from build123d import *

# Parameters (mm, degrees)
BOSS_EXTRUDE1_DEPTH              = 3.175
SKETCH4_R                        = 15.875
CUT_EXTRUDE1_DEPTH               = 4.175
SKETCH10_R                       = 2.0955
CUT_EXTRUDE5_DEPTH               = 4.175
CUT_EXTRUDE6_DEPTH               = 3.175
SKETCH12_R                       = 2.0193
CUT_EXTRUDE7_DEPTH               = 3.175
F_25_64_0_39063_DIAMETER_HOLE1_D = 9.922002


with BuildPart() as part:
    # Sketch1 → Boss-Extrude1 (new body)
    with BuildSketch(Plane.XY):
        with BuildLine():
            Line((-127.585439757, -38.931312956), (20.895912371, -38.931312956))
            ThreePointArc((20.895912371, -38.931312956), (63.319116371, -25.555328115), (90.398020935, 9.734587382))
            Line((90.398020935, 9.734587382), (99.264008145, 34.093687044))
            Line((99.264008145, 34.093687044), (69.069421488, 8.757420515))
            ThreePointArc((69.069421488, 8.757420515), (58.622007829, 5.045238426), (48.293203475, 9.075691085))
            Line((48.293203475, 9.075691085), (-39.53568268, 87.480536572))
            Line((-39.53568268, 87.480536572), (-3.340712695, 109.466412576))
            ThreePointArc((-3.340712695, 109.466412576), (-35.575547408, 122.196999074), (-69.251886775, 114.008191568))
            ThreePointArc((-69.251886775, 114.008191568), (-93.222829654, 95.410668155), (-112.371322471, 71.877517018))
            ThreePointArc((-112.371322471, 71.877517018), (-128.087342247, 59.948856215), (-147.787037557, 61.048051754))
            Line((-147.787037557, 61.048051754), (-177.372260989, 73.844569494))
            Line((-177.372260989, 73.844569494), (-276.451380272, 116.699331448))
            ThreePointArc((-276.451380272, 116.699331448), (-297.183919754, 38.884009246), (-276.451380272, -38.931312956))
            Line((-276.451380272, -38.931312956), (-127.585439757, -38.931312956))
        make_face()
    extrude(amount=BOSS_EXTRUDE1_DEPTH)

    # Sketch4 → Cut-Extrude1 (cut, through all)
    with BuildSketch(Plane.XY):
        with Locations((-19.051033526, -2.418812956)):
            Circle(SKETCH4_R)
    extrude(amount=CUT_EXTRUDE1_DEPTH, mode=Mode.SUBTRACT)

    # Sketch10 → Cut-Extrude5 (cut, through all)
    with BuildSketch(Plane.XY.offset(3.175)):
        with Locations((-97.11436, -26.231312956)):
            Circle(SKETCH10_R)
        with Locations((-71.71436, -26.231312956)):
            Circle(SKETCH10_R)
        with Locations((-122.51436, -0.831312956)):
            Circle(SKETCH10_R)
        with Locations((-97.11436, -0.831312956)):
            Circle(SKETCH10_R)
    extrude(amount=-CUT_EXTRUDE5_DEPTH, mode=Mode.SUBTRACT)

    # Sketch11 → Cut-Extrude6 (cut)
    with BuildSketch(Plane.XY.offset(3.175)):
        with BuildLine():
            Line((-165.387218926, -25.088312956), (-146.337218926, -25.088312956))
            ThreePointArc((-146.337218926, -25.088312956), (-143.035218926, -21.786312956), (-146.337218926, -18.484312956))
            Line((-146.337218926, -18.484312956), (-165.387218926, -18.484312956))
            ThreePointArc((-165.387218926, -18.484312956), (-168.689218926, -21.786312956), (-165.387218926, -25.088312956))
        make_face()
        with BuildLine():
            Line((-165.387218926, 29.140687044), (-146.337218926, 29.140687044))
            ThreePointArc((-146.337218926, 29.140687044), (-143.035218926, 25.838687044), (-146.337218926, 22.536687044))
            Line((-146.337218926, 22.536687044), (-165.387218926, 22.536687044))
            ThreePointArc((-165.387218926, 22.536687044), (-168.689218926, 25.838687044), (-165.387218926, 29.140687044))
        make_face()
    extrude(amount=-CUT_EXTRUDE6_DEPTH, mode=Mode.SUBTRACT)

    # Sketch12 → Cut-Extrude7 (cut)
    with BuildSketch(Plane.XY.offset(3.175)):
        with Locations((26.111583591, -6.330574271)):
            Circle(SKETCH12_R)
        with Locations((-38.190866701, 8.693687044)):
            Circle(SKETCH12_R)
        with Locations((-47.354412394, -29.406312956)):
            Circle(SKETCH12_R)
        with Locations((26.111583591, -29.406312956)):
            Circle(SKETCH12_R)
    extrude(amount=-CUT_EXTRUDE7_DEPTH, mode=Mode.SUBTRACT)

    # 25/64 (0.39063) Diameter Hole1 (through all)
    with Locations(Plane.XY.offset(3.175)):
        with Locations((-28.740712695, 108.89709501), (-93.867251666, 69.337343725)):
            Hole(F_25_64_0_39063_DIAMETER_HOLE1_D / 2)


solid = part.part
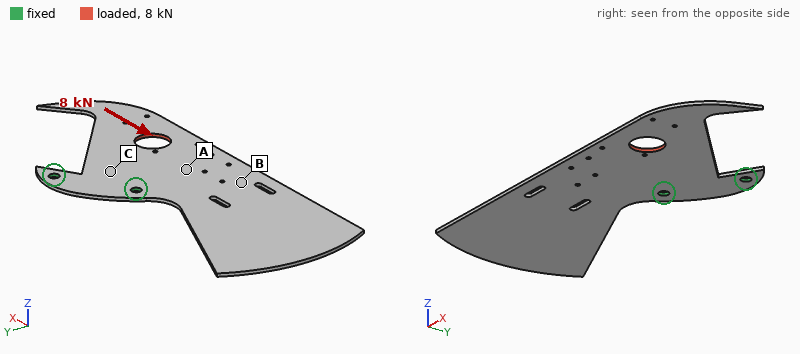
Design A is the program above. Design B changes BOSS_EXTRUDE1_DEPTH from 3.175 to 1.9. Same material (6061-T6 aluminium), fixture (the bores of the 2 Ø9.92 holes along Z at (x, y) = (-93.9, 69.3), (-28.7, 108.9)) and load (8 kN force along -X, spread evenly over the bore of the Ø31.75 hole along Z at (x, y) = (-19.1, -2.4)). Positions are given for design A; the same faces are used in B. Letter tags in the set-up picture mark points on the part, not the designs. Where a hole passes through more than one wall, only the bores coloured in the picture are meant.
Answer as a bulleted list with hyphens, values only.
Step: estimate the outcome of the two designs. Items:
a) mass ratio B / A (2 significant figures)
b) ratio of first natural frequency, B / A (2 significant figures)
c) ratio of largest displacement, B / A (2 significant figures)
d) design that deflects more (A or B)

- 0.60
- 0.60
- 1.7
- B
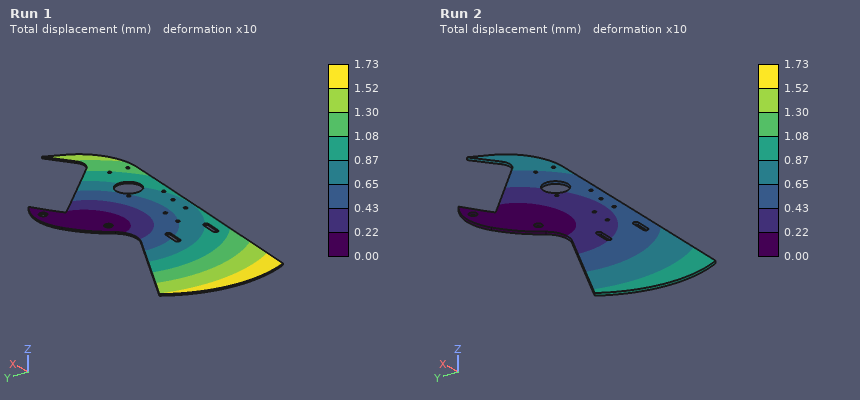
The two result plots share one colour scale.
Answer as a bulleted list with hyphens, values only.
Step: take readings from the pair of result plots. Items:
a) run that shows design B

- Run 1
